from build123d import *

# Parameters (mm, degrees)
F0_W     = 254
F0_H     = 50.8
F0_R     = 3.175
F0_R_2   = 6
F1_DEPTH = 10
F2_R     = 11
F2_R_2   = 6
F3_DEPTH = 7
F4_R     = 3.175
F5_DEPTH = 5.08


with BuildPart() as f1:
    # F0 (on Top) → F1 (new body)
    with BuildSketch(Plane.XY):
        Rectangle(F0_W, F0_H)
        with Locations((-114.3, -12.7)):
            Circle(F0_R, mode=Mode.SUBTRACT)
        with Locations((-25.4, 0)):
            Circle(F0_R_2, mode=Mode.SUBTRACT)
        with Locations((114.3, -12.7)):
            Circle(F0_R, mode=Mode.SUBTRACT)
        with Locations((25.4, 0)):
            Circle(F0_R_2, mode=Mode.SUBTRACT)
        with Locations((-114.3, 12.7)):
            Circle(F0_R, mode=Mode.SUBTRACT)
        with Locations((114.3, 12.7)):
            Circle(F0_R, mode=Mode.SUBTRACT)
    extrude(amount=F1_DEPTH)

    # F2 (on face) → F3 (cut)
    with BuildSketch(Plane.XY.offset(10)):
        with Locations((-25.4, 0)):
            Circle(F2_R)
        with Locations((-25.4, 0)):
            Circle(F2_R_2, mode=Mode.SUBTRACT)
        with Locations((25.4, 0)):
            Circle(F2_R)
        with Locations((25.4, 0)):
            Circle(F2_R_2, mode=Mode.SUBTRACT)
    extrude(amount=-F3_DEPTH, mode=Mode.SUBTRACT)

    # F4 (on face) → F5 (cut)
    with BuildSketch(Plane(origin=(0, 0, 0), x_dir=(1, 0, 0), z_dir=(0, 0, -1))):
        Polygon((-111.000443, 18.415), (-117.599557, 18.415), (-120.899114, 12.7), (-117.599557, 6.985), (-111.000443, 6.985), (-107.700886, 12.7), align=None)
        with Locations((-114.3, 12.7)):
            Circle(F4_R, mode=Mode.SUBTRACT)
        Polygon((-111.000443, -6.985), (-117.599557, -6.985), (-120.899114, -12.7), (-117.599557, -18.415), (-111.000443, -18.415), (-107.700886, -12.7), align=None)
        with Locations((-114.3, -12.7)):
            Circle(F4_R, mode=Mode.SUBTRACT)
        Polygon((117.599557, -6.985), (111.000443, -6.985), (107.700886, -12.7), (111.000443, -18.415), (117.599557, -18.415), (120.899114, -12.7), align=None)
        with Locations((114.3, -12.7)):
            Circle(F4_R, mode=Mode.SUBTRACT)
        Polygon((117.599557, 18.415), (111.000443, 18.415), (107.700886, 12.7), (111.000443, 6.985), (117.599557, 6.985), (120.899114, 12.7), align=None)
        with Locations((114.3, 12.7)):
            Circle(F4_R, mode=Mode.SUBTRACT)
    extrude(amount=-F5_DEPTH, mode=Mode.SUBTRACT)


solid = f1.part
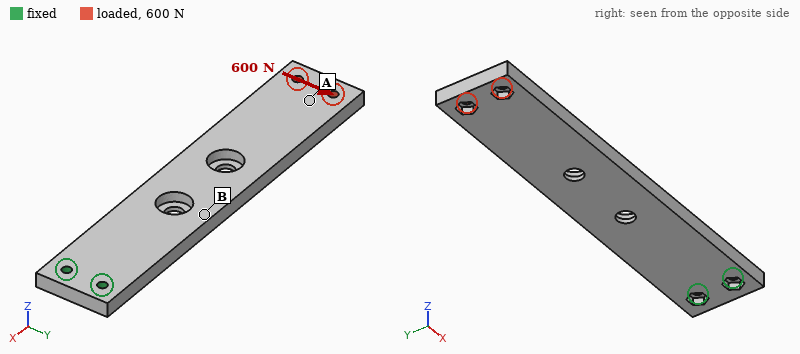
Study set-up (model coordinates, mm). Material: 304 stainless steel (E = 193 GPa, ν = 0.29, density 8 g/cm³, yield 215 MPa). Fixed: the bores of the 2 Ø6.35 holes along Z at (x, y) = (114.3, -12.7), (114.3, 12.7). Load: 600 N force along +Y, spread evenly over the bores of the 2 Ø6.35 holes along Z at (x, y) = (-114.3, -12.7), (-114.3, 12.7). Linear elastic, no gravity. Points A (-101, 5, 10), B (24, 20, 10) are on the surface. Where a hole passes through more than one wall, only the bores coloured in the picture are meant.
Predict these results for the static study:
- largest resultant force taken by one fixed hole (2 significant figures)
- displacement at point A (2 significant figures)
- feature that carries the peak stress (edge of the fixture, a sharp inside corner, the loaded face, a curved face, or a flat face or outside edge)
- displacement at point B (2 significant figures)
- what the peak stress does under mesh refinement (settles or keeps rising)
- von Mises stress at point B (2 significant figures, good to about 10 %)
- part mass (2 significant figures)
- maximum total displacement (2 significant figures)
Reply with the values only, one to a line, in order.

4.7 kN
0.14 mm
edge of the fixture
0.042 mm
keeps rising
17 MPa
960 g
0.17 mm
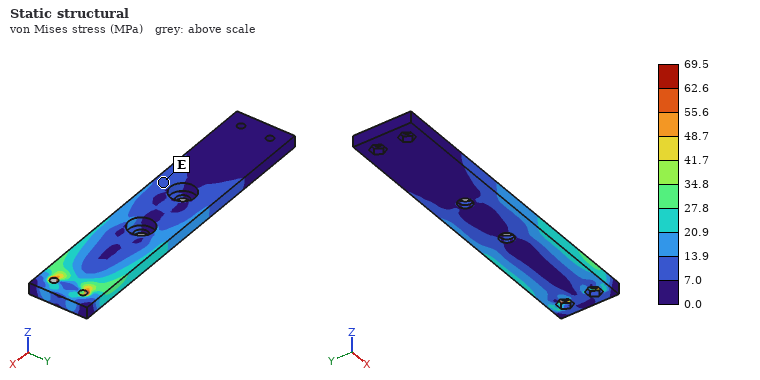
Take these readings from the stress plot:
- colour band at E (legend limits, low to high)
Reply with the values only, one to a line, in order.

7.0 to 13.9 MPa
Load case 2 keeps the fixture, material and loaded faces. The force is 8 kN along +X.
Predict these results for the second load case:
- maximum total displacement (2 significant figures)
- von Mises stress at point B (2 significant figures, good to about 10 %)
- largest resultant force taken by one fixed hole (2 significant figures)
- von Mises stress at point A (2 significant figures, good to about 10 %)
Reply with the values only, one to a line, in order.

0.81 mm
61 MPa
4.0 kN
39 MPa
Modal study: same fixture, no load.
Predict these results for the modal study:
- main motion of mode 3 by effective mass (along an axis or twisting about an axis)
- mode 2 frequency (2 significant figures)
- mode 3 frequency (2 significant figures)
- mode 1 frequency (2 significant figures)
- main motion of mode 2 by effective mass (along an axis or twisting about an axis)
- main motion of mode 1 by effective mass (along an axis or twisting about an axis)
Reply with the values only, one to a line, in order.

along Z
590 Hz
760 Hz
120 Hz
along Y
along Z
